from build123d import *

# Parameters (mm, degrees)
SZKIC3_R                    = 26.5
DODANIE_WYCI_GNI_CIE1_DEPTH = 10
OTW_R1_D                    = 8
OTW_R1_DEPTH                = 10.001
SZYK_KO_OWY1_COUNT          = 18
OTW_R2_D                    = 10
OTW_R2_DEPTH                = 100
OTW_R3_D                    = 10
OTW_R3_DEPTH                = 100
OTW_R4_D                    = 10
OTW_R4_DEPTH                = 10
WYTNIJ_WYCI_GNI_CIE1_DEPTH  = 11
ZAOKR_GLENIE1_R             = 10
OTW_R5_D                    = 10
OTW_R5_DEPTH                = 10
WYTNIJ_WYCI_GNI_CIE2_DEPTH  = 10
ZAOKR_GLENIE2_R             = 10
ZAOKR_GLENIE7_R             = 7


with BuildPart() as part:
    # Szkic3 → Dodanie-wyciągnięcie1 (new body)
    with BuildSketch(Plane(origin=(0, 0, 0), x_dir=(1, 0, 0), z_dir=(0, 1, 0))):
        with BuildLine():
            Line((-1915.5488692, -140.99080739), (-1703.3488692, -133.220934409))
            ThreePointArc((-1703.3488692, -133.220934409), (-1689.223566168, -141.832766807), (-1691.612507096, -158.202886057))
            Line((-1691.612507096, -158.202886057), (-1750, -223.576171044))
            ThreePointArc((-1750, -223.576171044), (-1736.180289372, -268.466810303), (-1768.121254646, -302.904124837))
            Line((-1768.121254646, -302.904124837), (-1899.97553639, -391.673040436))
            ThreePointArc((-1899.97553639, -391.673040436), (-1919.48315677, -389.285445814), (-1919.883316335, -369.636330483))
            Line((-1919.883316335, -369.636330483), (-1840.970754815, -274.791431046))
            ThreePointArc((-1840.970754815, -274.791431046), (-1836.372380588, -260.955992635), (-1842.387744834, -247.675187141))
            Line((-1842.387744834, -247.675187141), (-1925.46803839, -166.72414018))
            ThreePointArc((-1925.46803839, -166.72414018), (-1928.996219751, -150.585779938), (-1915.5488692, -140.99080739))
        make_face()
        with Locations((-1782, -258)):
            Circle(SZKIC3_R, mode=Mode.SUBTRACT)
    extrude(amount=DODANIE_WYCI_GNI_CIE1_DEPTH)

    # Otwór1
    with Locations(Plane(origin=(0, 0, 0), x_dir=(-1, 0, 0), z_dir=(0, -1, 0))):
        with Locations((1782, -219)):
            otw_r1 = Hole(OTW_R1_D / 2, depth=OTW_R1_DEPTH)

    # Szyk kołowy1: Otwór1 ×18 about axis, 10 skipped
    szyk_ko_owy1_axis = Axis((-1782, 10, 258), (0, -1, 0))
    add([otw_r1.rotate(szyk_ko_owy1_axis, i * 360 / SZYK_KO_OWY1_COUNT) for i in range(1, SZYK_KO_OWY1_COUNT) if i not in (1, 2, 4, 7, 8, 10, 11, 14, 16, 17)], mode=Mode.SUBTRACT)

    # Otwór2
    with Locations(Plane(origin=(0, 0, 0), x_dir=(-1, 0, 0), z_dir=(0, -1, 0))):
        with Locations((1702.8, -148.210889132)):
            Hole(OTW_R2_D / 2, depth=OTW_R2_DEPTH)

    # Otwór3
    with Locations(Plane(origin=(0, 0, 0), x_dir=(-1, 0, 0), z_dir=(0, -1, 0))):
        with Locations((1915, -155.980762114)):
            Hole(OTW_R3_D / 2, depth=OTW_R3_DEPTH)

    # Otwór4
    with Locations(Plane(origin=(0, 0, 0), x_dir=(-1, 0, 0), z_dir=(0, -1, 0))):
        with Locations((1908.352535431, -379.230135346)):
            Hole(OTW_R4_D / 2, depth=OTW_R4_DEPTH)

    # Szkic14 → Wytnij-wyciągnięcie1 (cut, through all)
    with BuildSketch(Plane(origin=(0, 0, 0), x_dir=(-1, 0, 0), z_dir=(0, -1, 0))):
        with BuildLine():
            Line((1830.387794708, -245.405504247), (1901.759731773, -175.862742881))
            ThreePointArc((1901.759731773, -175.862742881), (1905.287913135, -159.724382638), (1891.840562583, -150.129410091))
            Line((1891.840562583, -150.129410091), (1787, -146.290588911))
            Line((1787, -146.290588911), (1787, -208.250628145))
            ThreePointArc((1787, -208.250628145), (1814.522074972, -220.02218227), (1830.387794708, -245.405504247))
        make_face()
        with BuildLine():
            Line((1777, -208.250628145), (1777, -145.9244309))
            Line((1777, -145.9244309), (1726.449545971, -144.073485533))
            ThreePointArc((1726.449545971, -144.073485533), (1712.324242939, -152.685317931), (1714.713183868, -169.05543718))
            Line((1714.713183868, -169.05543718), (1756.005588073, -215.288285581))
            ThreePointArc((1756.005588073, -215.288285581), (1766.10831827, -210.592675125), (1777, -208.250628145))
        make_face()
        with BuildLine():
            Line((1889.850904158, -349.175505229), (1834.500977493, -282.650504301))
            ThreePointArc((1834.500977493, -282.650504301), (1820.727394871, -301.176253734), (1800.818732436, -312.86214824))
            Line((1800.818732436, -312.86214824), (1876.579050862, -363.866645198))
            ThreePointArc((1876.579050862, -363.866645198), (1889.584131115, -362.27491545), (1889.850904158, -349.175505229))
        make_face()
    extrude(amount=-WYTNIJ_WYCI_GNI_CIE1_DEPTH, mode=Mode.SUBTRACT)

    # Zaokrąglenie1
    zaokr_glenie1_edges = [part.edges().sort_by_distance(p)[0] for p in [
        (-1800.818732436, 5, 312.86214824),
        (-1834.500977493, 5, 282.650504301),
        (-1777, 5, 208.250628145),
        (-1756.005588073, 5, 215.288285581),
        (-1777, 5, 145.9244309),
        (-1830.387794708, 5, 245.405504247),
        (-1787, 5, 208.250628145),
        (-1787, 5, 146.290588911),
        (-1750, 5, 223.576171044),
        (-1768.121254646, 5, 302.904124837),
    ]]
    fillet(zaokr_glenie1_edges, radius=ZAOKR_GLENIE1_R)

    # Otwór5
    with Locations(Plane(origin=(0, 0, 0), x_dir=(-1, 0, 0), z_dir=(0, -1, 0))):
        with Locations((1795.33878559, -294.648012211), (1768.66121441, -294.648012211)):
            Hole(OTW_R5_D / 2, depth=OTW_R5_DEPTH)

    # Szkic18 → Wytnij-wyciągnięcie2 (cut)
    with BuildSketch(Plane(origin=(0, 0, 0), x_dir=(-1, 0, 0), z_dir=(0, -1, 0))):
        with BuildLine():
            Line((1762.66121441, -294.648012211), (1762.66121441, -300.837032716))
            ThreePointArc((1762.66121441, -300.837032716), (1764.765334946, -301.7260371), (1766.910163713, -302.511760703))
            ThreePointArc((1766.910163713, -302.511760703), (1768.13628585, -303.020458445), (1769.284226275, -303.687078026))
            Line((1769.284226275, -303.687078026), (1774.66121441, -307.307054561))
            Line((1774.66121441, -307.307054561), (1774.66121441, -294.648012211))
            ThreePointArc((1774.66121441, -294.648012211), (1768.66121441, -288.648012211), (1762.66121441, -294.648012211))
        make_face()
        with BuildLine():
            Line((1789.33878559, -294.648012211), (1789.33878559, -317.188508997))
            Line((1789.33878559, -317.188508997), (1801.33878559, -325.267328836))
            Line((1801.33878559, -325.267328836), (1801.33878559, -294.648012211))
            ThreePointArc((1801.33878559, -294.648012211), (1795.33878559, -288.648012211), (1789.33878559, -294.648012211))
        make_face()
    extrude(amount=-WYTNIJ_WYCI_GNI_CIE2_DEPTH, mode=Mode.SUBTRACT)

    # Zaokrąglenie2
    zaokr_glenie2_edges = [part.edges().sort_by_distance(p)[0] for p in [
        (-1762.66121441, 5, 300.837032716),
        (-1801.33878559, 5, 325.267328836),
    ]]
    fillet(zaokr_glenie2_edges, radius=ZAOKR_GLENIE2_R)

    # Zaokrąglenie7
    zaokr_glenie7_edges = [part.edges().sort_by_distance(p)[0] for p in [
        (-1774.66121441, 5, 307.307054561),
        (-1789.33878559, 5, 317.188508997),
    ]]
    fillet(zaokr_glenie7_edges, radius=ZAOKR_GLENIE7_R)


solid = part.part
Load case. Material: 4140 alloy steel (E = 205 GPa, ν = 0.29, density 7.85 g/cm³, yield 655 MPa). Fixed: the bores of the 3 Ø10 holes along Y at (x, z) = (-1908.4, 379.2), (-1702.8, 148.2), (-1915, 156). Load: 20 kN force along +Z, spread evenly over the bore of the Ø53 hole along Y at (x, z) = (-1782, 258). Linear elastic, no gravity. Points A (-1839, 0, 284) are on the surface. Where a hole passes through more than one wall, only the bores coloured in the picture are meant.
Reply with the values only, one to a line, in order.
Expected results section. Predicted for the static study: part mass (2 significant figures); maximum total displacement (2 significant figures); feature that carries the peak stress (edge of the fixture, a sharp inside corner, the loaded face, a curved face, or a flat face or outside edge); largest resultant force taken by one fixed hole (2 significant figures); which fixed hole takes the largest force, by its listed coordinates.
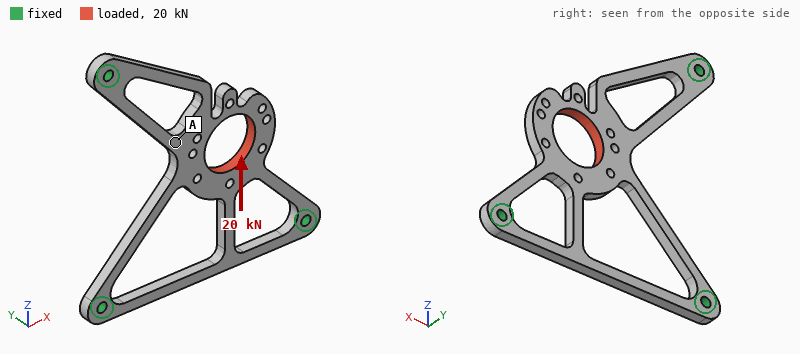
1.1 kg
0.25 mm
a curved face
12 kN
(-1915, 156)
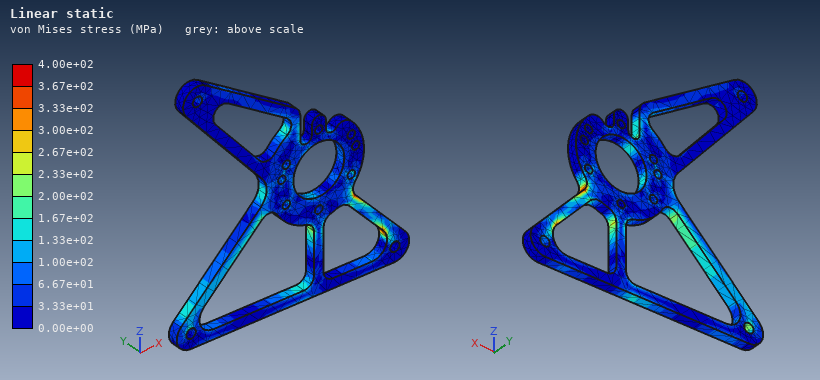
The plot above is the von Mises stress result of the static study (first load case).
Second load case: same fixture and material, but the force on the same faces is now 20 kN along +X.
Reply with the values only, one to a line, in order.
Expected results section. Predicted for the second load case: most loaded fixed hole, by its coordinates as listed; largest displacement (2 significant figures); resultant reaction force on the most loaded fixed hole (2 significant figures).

(-1915, 156)
0.20 mm
13 kN
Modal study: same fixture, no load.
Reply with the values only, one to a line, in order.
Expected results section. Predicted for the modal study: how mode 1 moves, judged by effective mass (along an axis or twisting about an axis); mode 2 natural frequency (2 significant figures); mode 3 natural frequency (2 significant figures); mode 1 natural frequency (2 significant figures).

along Y
990 Hz
1200 Hz
420 Hz
